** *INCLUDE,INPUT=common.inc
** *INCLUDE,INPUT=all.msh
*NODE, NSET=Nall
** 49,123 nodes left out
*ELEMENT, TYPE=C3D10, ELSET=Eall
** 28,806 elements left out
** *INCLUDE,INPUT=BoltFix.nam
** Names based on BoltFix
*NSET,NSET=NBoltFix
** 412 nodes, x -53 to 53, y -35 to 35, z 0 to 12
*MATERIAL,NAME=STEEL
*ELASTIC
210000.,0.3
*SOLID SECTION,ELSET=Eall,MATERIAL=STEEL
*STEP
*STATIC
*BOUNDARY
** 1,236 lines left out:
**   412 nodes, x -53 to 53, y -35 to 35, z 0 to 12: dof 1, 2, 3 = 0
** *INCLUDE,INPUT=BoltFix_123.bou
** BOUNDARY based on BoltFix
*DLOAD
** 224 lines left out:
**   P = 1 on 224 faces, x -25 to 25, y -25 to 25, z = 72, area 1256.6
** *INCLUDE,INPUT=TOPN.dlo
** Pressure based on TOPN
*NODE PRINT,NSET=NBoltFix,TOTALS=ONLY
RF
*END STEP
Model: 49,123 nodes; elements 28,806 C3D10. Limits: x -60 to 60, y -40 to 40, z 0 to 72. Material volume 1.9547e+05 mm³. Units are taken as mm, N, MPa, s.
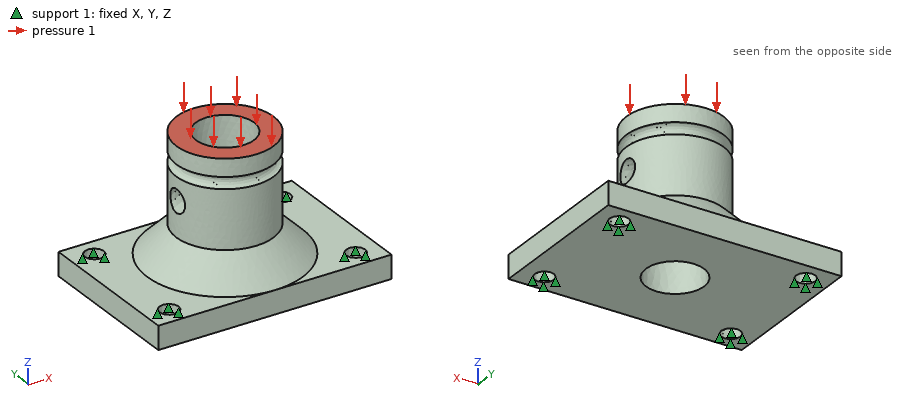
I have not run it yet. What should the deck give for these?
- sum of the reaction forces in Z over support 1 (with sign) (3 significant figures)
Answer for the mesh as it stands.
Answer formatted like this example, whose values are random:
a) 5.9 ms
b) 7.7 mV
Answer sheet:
a) 1260 N
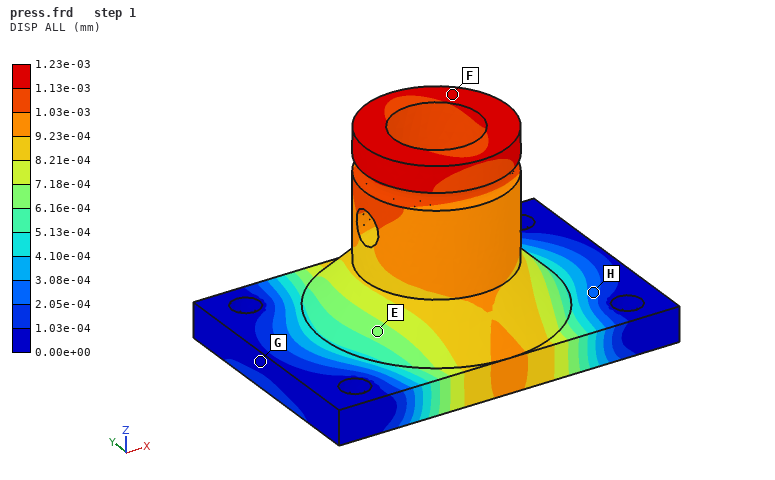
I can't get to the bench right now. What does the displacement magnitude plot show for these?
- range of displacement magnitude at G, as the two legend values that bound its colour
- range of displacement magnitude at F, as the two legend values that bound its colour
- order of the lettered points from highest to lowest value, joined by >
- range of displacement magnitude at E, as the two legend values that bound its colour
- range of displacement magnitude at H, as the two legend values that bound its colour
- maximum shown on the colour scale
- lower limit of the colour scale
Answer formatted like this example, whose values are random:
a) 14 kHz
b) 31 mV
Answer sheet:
a) 0.00e+00 to 1.03e-04 mm
b) 1.13e-03 to 1.23e-03 mm
c) F > E > H > G
d) 6.16e-04 to 7.18e-04 mm
e) 2.05e-04 to 3.08e-04 mm
f) 1.23e-03 mm
g) 0.00e+00 mm
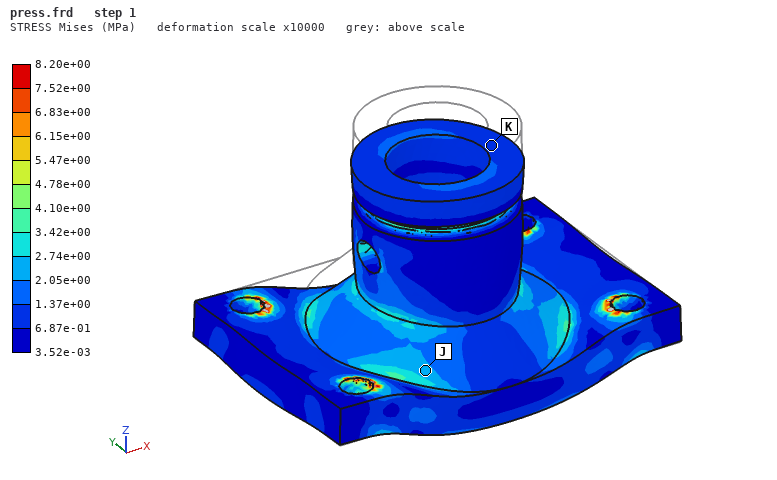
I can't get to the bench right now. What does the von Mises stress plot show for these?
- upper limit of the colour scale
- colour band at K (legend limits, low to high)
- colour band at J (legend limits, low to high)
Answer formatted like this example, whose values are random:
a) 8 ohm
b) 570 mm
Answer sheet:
a) 8.20e+00 MPa
b) 6.87e-01 to 1.37e+00 MPa
c) 2.05e+00 to 2.74e+00 MPa
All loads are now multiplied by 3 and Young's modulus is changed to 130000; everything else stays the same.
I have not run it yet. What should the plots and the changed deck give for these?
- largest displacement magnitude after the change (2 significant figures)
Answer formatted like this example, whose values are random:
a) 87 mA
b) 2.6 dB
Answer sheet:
a) 0.0060 mm
